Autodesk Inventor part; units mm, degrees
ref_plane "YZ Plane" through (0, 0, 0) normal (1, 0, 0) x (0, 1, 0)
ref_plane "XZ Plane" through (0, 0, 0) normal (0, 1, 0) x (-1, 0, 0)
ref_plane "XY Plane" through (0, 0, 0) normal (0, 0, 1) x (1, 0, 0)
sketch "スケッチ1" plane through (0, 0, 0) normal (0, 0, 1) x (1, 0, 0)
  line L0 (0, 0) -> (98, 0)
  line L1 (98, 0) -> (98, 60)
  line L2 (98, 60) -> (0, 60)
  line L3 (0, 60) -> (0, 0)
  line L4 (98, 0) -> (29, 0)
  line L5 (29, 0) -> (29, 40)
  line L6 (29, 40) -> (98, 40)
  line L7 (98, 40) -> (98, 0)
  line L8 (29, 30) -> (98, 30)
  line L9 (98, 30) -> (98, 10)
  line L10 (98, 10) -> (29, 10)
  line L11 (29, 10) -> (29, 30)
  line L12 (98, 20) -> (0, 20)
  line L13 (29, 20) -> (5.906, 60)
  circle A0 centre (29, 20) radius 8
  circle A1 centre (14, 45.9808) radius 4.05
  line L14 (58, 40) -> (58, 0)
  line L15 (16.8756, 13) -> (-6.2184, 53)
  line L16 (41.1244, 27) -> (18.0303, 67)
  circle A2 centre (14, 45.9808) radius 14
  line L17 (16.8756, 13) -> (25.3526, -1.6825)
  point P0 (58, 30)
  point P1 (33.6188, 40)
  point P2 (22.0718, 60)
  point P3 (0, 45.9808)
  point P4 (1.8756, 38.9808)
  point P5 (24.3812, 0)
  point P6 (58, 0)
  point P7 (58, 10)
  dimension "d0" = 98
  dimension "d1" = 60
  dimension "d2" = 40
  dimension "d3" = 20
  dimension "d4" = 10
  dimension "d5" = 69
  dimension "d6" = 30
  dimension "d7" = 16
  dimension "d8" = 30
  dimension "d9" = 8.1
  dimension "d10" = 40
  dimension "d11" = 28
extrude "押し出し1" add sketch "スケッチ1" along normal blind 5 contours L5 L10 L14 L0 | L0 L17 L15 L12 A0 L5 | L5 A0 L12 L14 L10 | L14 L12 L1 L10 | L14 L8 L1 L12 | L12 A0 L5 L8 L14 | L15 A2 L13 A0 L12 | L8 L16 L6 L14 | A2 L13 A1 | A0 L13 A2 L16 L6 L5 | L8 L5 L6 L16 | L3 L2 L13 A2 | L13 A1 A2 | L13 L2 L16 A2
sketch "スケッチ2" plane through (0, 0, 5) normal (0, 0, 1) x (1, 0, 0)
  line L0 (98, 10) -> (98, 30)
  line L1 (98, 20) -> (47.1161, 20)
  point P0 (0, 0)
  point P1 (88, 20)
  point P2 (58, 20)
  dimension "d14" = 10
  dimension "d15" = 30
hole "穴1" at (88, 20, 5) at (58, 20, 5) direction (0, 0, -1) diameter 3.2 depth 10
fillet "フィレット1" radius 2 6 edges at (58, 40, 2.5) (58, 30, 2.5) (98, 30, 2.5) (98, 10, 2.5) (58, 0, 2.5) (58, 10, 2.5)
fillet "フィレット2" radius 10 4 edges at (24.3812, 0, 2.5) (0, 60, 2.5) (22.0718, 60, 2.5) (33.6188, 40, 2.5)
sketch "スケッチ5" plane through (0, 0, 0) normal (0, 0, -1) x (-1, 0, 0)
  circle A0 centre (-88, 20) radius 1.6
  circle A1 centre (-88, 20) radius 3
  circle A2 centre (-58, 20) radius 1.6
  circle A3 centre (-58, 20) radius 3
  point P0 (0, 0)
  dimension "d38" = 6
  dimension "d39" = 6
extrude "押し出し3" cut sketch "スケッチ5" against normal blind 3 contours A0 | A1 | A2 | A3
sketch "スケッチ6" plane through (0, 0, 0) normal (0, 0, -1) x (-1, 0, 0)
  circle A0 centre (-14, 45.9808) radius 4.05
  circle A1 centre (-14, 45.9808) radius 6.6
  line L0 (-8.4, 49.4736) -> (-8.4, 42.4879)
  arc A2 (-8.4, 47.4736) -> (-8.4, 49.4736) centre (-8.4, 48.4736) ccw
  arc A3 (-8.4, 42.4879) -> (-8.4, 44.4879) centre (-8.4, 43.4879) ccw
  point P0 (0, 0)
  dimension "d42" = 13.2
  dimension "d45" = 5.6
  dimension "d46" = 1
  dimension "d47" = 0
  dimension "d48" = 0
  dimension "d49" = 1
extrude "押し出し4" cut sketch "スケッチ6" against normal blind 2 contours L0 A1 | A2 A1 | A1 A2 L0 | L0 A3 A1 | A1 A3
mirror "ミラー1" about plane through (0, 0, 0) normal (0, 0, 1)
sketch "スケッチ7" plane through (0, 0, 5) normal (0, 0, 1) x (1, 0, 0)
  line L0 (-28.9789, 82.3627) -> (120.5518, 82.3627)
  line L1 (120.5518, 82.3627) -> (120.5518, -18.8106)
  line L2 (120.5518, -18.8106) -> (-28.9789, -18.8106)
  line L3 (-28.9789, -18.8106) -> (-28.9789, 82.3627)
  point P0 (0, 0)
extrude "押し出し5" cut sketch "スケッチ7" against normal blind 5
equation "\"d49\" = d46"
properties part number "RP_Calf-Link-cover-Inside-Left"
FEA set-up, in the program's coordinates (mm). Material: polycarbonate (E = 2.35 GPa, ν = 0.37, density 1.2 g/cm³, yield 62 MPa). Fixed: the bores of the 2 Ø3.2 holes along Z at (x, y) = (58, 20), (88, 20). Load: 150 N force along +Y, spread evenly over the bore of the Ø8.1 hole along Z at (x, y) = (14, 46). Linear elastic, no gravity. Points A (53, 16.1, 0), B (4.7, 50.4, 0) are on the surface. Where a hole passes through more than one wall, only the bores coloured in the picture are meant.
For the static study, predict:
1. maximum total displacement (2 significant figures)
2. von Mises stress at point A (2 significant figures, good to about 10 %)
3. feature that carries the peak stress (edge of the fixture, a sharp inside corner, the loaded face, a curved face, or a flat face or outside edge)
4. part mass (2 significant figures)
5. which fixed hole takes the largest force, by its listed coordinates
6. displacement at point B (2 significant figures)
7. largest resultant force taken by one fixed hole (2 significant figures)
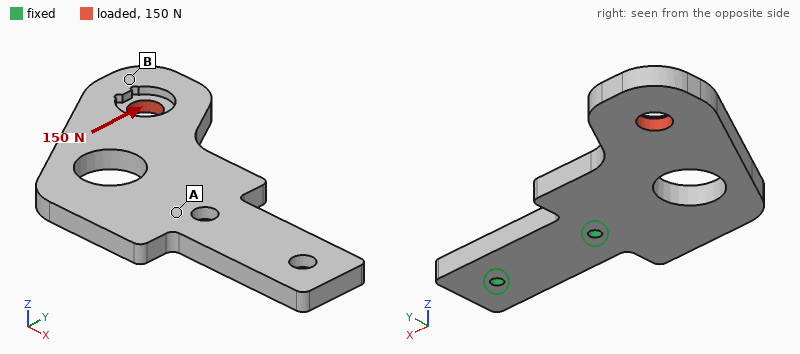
1.3 mm
7.7 MPa
edge of the fixture
17 g
(58, 20)
1.2 mm
350 N
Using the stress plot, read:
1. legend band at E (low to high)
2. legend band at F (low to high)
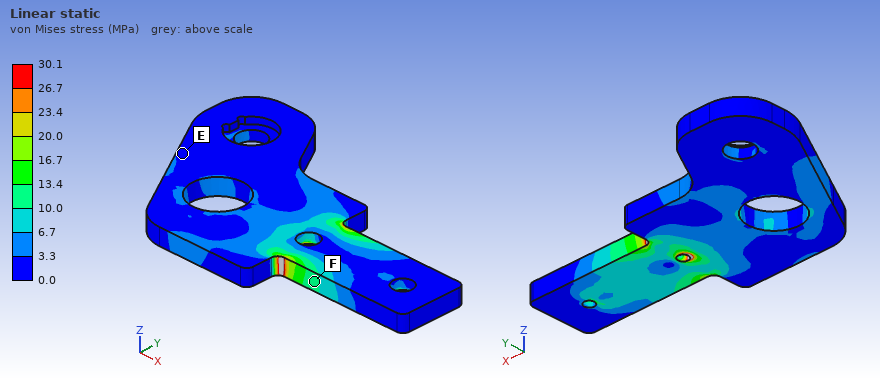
0.0 to 3.3 MPa
10.0 to 13.4 MPa
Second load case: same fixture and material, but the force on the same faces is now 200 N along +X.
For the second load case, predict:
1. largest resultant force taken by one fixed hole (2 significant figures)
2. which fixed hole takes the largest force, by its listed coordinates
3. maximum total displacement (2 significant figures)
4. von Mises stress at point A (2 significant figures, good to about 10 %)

220 N
(58, 20)
1.2 mm
5.5 MPa
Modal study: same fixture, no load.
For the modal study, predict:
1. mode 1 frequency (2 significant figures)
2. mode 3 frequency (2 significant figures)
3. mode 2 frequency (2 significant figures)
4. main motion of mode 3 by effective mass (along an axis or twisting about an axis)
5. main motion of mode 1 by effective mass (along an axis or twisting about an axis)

230 Hz
750 Hz
560 Hz
along Y
along Z
